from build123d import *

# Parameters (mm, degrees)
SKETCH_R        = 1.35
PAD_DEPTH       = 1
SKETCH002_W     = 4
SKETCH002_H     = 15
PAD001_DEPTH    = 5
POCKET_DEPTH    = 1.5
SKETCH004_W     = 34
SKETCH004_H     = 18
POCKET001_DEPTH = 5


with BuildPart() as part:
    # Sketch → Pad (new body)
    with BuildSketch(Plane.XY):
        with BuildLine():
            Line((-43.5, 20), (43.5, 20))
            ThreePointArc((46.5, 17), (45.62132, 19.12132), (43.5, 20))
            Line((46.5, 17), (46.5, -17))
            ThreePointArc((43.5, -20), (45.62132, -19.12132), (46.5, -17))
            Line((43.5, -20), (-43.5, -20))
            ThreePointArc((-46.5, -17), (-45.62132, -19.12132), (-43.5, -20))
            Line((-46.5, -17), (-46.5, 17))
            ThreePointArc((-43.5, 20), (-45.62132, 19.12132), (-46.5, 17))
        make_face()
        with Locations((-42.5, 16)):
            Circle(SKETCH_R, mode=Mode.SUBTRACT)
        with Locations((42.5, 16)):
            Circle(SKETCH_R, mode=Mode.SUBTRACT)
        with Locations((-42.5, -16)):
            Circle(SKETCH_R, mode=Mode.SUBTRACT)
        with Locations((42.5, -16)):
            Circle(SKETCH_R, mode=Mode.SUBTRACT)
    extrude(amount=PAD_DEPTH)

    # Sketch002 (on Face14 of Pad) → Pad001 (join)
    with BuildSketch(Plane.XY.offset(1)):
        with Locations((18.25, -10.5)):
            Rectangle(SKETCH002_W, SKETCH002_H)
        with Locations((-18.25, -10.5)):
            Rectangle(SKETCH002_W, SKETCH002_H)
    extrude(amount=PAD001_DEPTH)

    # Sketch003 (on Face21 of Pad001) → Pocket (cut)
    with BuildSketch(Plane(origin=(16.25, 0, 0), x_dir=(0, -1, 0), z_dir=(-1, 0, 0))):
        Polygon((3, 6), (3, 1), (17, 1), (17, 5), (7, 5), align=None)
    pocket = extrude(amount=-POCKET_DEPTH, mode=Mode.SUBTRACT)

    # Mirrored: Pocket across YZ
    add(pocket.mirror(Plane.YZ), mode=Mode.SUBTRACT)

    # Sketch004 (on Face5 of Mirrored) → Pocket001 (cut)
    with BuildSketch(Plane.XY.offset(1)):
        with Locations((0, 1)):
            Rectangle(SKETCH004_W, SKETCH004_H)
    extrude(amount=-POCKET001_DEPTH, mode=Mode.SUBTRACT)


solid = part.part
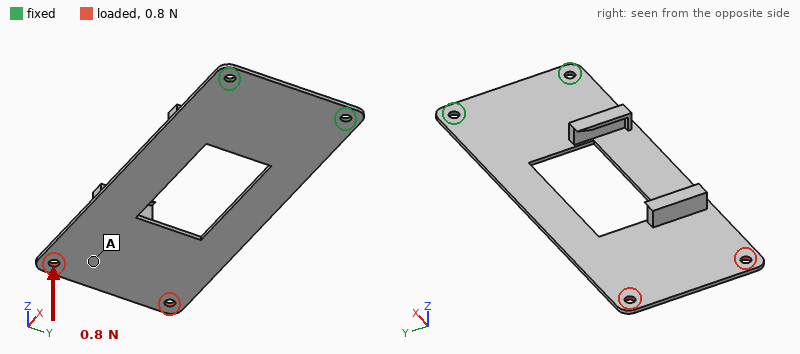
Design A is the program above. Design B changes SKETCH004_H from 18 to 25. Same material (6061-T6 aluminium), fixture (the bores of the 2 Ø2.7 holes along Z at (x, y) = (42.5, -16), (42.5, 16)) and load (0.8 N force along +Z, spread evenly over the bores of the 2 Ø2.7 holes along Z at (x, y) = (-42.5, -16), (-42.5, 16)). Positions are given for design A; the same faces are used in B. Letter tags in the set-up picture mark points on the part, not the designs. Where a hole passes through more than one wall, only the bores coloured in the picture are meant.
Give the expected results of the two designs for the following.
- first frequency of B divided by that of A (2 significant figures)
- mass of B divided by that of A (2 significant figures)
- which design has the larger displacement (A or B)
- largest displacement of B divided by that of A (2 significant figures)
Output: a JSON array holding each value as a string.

["0.93", "0.93", "B", "1.2"]
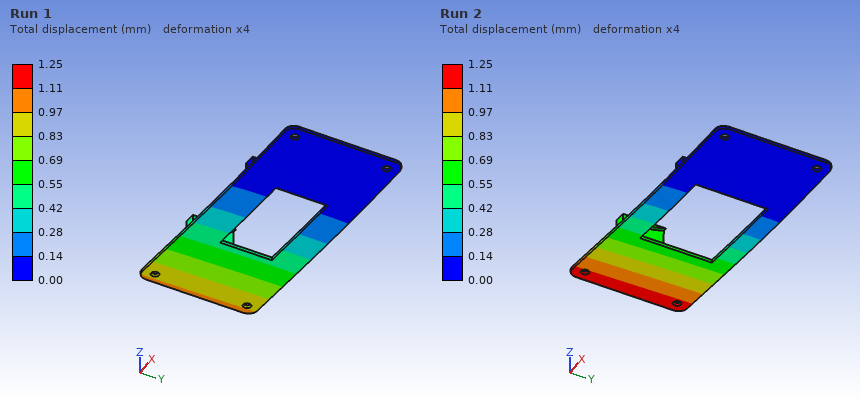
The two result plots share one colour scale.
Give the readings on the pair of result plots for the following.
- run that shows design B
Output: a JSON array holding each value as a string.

["Run 2"]
